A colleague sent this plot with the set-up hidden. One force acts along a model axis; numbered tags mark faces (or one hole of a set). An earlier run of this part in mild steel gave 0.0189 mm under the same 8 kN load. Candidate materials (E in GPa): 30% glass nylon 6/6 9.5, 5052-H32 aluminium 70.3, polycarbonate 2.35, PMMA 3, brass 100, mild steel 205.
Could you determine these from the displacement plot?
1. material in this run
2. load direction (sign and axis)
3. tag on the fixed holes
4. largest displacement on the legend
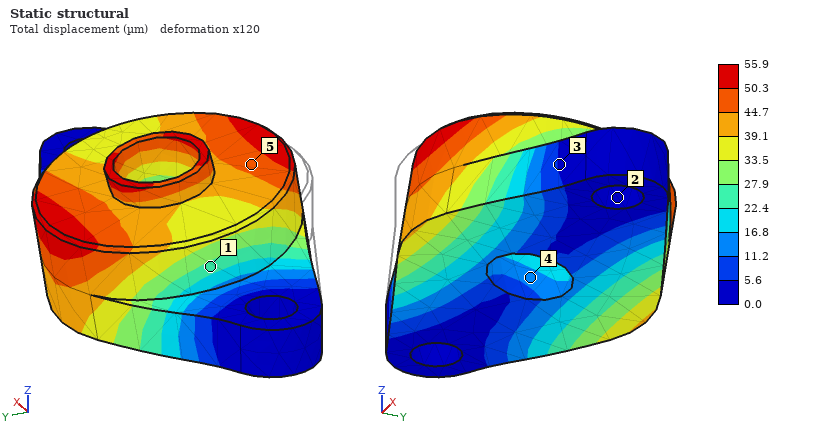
5052-H32 aluminium
+Y
2
55.9 µm
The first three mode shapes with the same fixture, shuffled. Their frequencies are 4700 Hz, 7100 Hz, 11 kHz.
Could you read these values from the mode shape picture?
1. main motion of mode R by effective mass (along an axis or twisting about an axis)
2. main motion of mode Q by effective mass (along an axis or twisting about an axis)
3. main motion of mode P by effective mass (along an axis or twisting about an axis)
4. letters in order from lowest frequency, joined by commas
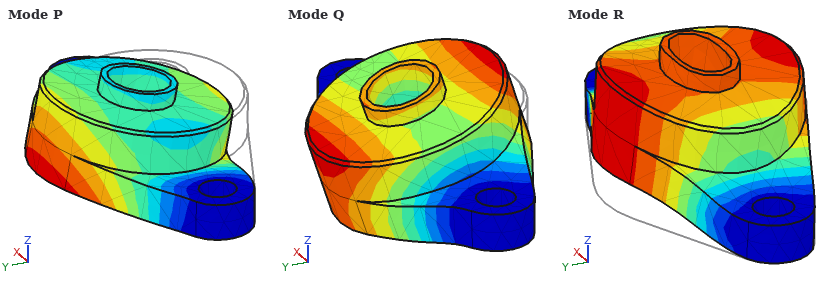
along Z
along Y
along Y
Q, R, P
